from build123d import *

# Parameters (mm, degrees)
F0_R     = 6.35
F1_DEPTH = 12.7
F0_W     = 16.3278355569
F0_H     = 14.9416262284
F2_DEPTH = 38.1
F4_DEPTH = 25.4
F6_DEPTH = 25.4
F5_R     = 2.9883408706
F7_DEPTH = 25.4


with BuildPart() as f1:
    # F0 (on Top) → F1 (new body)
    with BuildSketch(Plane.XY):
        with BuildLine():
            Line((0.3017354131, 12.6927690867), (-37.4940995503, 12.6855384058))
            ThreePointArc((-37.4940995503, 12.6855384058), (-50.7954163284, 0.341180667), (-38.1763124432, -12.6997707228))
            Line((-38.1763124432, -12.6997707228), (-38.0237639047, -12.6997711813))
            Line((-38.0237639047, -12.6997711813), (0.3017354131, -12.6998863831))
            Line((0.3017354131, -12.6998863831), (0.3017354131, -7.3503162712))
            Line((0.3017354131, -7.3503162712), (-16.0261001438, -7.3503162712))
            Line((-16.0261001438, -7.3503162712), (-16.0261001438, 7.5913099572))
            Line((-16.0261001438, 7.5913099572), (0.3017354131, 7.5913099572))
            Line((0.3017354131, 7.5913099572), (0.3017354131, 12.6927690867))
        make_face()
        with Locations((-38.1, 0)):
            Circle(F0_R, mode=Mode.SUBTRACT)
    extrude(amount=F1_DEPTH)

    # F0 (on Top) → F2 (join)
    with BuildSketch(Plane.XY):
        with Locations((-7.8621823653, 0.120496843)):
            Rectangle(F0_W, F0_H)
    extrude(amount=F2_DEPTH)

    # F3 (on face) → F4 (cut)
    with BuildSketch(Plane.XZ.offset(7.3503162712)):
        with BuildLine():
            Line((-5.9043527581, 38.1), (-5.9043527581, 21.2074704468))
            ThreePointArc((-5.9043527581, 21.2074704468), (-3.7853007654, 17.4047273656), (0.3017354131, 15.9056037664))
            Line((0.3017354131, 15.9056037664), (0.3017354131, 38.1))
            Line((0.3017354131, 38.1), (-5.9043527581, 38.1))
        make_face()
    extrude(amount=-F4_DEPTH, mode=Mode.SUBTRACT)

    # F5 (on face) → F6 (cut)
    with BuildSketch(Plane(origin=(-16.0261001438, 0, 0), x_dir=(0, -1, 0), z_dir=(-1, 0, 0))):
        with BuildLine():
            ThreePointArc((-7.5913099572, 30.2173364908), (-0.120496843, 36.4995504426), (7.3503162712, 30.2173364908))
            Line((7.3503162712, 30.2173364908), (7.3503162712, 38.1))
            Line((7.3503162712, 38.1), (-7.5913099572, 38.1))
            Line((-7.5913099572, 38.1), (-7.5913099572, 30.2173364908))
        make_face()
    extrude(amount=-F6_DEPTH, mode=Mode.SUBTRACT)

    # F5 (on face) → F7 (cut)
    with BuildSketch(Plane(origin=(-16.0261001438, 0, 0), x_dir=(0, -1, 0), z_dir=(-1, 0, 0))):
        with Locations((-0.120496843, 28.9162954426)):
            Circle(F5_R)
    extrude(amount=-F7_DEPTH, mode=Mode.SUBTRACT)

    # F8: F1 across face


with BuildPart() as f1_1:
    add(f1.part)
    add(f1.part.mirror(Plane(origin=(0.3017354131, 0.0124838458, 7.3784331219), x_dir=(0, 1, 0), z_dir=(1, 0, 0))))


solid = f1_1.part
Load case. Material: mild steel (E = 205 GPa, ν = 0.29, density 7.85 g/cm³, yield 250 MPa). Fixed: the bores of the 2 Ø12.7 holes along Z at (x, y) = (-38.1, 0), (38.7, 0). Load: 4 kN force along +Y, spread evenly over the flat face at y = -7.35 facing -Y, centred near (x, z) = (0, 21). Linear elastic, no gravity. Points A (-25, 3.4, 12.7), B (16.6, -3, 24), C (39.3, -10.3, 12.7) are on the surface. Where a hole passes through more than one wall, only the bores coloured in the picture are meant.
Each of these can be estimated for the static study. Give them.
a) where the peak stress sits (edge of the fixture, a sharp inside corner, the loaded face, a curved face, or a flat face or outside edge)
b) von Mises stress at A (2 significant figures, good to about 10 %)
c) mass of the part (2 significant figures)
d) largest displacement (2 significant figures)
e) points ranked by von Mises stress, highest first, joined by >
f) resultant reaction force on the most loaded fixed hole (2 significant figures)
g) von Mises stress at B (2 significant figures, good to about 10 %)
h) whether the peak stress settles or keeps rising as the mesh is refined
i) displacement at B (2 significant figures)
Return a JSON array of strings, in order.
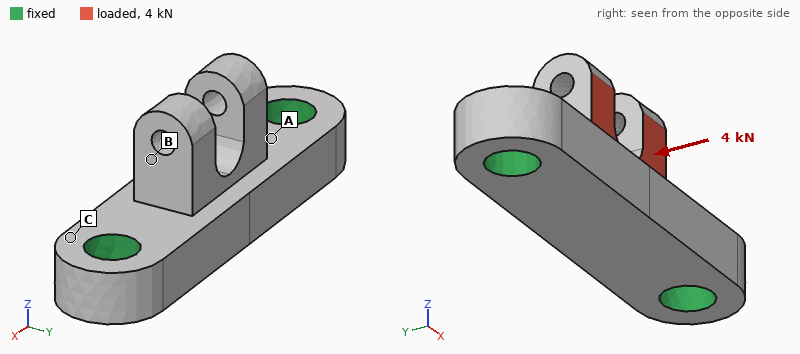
["edge of the fixture", "52 MPa", "270 g", "27 µm", "A > B > C", "2.0 kN", "13 MPa", "keeps rising", "17 µm"]
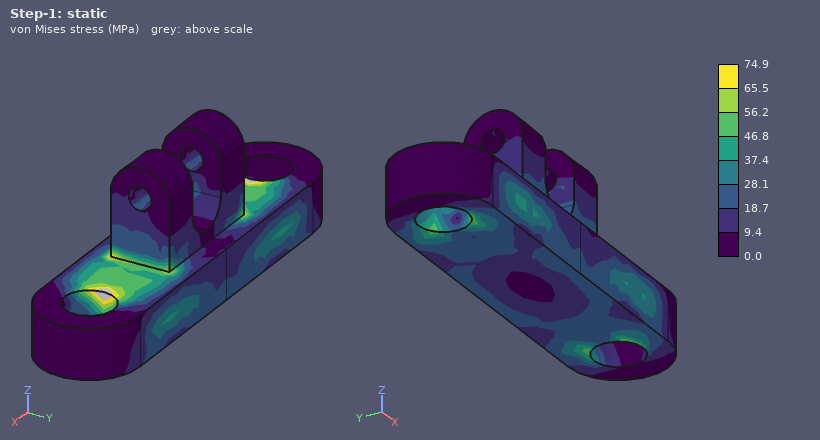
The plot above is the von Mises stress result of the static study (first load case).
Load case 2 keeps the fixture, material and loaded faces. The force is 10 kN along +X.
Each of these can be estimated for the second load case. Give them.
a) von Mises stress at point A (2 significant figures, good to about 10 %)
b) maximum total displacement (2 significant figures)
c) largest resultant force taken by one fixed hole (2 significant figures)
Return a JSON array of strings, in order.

["22 MPa", "28 µm", "5.8 kN"]
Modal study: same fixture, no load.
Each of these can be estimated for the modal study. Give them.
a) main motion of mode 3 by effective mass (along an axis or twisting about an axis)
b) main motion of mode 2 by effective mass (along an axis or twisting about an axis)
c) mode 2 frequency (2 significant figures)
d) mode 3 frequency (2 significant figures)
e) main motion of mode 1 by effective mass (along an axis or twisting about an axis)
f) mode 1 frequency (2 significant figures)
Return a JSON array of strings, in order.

["along X", "along Z", "10 kHz", "14 kHz", "along Y", "8500 Hz"]
